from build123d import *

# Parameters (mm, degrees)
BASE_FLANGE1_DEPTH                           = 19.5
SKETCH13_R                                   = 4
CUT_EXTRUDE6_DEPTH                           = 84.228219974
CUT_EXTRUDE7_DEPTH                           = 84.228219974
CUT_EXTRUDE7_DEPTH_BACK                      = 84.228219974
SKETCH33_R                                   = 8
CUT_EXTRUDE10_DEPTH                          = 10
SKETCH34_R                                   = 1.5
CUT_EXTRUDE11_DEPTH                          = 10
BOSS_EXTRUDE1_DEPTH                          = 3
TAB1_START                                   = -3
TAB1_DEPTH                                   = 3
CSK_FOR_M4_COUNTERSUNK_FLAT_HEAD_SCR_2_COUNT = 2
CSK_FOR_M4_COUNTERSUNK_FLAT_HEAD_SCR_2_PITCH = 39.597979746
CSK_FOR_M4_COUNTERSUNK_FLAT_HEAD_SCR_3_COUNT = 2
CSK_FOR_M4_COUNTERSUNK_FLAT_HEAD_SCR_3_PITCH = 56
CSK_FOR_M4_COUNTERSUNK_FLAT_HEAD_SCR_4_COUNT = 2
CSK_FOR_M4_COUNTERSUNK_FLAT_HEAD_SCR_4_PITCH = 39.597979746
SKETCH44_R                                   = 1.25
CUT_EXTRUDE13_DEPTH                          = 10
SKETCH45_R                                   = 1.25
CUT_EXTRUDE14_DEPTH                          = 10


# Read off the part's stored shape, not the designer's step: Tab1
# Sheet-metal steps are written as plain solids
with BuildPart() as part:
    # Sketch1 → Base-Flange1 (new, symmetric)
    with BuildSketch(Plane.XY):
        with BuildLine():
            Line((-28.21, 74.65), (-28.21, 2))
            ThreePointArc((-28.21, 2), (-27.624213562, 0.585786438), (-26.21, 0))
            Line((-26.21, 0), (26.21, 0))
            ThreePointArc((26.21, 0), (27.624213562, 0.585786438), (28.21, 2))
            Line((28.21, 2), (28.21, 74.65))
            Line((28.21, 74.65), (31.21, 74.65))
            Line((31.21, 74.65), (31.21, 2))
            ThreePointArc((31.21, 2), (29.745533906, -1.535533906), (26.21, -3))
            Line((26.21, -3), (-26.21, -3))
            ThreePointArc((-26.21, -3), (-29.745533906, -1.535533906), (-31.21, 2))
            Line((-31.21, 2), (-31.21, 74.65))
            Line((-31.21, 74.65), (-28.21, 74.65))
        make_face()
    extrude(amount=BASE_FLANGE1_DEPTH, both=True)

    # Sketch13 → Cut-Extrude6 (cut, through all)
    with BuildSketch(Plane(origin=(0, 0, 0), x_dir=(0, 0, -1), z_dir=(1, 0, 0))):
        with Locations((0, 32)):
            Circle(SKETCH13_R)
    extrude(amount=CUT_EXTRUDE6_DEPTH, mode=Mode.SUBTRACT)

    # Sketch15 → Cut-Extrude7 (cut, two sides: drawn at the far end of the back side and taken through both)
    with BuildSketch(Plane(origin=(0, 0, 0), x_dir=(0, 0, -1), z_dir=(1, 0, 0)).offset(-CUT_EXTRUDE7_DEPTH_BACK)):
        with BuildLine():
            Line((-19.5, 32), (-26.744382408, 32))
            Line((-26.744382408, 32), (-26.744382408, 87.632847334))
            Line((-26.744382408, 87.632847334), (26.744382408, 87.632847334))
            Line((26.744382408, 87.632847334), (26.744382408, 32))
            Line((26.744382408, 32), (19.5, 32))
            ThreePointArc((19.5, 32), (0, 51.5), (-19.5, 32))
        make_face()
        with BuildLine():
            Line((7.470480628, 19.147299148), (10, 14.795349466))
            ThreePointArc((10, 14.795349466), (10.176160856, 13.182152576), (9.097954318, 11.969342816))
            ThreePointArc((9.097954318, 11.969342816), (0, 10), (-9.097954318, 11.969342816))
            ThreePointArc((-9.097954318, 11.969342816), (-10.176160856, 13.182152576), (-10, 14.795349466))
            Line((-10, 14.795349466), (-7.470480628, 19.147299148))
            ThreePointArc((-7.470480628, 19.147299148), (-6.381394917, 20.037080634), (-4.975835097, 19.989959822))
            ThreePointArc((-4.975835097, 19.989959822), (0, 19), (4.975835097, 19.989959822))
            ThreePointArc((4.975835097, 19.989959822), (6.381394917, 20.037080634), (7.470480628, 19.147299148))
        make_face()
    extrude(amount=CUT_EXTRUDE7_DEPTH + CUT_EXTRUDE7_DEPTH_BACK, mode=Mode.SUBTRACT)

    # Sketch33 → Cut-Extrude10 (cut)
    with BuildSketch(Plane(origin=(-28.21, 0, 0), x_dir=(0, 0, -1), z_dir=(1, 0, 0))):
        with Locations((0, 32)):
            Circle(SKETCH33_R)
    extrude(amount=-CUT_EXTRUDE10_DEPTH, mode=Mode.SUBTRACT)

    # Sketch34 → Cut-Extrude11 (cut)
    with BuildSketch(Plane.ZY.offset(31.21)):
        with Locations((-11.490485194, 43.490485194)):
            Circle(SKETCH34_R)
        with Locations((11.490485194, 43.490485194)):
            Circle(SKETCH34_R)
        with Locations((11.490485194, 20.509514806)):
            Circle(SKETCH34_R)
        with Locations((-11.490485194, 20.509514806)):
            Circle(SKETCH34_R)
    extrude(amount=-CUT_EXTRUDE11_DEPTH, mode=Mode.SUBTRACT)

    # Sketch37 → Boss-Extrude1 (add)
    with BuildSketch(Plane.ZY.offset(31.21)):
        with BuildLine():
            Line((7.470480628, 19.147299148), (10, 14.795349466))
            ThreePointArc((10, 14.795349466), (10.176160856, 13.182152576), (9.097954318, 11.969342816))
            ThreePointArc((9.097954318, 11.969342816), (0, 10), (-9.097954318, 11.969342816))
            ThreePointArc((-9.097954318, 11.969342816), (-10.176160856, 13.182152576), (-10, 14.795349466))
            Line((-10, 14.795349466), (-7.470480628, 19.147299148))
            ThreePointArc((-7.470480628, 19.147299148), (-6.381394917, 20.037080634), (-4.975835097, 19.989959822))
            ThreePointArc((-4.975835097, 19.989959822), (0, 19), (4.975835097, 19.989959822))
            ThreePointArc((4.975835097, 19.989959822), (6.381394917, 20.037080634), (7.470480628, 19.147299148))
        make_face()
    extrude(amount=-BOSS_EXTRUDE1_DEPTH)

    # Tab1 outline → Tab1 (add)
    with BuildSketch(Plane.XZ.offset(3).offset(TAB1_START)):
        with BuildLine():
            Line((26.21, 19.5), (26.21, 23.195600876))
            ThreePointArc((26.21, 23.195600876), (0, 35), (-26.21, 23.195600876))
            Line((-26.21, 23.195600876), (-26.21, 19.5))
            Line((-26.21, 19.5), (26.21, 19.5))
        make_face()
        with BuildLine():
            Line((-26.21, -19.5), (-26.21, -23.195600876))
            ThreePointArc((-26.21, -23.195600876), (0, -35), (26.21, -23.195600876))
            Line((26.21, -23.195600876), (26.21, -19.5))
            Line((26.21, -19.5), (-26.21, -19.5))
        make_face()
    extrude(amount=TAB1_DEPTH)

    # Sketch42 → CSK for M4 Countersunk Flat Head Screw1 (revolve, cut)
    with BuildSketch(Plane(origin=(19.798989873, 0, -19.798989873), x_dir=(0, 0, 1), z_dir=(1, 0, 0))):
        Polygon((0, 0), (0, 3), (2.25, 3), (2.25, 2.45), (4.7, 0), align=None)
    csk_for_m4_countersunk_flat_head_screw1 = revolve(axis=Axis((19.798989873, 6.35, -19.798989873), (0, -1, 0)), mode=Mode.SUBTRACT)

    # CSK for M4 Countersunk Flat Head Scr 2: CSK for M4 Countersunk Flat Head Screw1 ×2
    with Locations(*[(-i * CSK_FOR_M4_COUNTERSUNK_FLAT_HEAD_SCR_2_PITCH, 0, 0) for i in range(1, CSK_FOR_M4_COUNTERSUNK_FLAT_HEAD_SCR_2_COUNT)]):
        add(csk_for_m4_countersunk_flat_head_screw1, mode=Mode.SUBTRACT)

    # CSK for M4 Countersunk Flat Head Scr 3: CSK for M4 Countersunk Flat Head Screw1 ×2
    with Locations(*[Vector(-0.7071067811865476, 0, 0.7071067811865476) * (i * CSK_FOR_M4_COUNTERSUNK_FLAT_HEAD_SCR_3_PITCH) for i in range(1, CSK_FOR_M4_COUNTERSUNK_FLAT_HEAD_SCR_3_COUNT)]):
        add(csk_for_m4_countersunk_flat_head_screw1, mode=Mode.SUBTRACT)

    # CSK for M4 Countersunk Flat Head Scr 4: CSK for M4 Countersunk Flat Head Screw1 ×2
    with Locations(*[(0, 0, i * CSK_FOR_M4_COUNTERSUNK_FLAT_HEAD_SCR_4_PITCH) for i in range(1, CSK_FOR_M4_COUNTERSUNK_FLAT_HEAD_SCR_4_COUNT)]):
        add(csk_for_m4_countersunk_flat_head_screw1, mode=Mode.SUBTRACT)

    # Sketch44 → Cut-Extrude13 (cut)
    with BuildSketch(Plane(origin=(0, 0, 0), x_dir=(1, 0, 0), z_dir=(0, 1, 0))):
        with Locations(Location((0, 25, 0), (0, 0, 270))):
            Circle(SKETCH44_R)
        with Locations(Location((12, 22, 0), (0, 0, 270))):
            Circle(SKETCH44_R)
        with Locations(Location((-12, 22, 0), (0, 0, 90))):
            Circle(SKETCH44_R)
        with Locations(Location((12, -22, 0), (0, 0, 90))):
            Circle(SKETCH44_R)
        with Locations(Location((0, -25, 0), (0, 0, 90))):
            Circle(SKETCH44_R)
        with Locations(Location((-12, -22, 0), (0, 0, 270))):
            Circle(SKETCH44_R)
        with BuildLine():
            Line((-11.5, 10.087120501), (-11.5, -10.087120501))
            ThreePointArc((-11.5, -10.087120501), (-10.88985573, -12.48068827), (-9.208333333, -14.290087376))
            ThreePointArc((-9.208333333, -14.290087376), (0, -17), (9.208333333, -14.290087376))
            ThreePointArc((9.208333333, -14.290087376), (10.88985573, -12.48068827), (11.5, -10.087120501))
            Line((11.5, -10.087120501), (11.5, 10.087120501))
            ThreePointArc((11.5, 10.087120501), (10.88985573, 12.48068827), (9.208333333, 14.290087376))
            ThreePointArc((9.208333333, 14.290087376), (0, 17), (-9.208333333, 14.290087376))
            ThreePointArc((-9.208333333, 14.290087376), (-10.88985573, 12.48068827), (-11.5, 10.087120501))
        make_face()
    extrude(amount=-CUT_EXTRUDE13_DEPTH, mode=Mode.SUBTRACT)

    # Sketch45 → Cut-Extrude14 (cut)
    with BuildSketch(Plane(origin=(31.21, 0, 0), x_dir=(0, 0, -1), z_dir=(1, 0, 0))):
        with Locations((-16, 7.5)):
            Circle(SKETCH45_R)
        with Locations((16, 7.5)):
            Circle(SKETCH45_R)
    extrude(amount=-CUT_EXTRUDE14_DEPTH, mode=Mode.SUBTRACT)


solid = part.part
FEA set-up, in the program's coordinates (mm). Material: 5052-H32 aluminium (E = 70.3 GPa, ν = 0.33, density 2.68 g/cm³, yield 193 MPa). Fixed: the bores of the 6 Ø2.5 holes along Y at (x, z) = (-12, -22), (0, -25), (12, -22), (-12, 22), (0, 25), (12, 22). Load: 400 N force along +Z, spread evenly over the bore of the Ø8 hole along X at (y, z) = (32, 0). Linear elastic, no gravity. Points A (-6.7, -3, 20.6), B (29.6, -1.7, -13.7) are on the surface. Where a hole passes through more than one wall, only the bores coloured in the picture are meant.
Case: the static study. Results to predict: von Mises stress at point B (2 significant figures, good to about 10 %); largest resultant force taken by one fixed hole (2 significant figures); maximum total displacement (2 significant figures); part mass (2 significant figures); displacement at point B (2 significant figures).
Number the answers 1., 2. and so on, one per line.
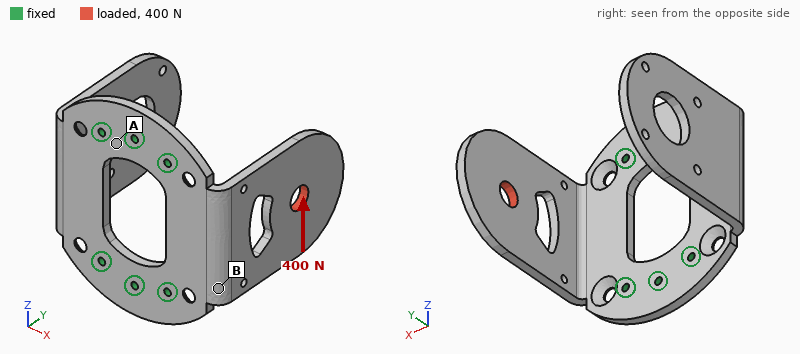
1. 77 MPa
2. 490 N
3. 0.45 mm
4. 48 g
5. 0.11 mm
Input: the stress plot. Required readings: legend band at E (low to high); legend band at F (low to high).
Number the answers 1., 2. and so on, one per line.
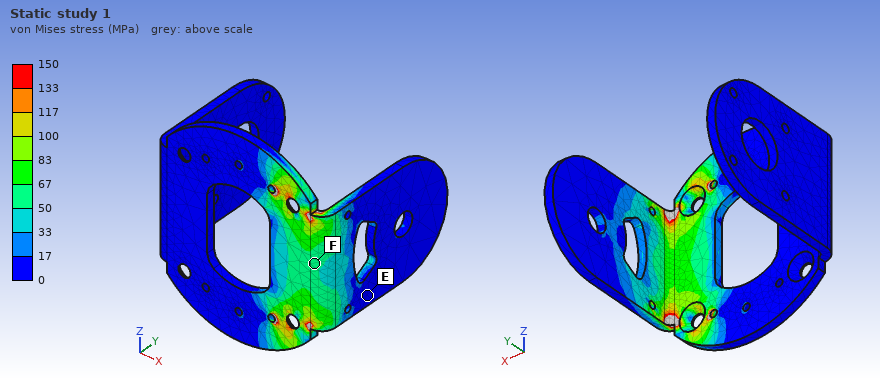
1. 0 to 17 MPa
2. 50 to 67 MPa
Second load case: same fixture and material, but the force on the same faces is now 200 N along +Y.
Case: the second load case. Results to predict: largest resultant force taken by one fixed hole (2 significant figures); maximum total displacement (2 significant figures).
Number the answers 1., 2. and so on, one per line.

1. 160 N
2. 0.39 mm
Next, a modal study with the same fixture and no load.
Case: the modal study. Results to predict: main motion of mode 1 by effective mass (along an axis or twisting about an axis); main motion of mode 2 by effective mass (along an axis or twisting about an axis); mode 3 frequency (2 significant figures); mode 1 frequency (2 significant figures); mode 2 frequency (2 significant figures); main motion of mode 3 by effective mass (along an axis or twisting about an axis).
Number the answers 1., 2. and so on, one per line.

1. along X
2. along X
3. 1700 Hz
4. 580 Hz
5. 660 Hz
6. along Z
